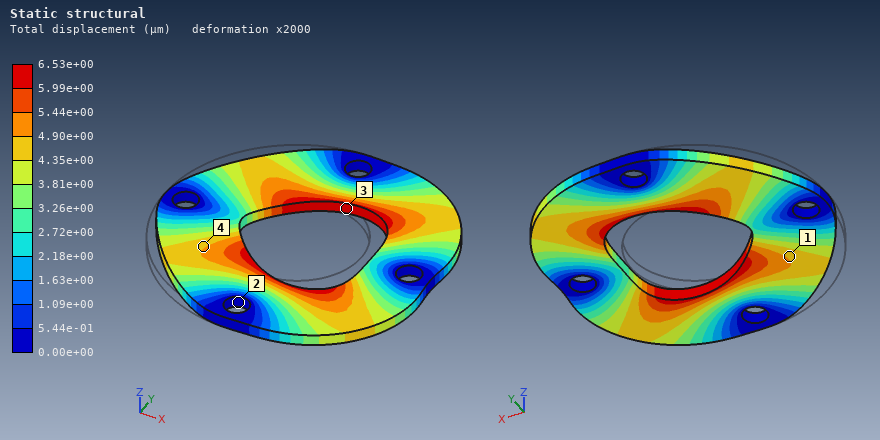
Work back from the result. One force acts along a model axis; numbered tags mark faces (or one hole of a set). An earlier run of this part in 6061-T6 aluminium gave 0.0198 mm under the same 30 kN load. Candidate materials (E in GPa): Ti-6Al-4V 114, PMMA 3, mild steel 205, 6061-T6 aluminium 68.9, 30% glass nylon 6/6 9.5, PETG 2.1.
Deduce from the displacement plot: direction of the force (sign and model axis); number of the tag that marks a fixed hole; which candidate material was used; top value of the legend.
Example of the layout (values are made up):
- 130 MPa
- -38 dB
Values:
- +X
- 2
- mild steel
- 6.53e+00 µm
